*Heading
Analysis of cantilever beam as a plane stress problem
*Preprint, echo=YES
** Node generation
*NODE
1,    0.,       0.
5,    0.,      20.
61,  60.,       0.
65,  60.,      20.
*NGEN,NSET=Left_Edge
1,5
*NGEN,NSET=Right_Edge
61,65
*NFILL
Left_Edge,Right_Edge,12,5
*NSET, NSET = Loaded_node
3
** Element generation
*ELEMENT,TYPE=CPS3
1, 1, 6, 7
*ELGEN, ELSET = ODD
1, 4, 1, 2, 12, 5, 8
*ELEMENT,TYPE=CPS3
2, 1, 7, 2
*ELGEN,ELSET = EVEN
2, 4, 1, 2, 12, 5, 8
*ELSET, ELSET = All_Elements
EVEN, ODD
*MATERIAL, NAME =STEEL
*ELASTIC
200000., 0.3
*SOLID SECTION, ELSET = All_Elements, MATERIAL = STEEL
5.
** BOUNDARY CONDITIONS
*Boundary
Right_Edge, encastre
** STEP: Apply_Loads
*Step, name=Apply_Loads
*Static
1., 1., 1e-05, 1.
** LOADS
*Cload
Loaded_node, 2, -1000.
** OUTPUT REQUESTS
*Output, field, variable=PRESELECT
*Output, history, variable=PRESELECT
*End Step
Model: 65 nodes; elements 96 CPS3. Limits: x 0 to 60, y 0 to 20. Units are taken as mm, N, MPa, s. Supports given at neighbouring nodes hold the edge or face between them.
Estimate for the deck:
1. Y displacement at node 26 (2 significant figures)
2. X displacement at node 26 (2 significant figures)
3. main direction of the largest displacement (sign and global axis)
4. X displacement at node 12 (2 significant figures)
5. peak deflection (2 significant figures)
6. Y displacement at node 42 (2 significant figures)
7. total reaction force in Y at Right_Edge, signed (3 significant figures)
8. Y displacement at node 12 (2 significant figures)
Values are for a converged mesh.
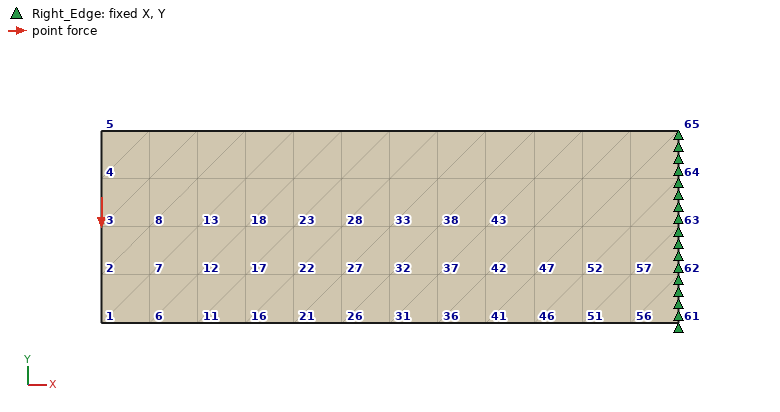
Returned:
-0.050 mm
0.022 mm
-Y
0.013 mm
0.12 mm
-0.019 mm
1000 N
-0.088 mm
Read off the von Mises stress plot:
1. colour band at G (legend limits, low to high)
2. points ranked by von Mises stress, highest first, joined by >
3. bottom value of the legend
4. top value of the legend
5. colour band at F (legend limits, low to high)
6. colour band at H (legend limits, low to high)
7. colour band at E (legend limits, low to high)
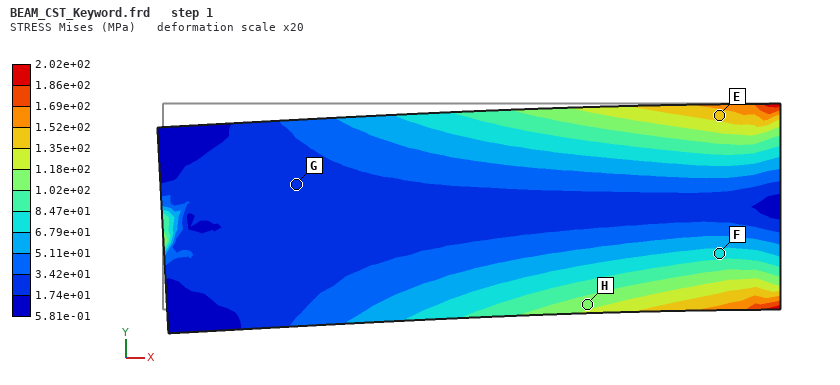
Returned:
1.74e+01 to 3.42e+01 MPa
E > H > F > G
5.81e-01 MPa
2.02e+02 MPa
6.79e+01 to 8.47e+01 MPa
1.02e+02 to 1.18e+02 MPa
1.35e+02 to 1.52e+02 MPa
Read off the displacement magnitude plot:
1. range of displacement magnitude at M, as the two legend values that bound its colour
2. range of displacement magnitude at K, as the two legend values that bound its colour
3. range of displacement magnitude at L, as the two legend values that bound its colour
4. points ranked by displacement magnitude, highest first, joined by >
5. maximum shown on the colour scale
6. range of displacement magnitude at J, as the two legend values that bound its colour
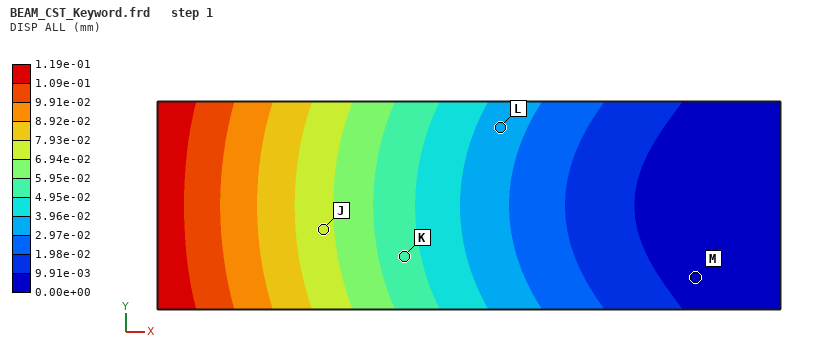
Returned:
0.00e+00 to 9.91e-03 mm
4.95e-02 to 5.95e-02 mm
2.97e-02 to 3.96e-02 mm
J > K > L > M
1.19e-01 mm
6.94e-02 to 7.93e-02 mm
